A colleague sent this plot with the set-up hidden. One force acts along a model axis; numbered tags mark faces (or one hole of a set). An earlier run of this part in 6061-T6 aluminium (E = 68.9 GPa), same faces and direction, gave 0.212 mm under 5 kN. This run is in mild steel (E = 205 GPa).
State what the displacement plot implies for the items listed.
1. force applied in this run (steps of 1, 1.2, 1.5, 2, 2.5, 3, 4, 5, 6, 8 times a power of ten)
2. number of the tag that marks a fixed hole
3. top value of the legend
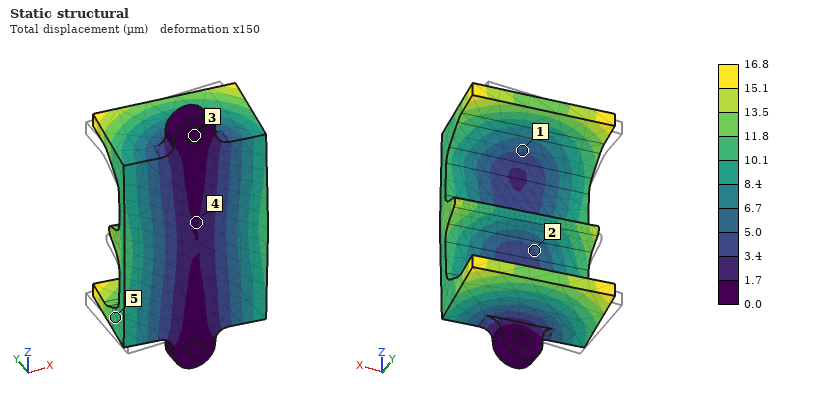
1.2 kN
3
16.8 µm
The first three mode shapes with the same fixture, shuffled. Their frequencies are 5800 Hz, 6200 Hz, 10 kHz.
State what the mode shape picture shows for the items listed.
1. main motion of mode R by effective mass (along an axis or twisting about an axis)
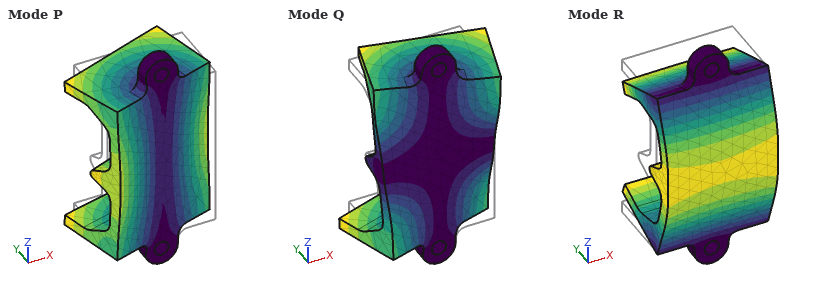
along Y
